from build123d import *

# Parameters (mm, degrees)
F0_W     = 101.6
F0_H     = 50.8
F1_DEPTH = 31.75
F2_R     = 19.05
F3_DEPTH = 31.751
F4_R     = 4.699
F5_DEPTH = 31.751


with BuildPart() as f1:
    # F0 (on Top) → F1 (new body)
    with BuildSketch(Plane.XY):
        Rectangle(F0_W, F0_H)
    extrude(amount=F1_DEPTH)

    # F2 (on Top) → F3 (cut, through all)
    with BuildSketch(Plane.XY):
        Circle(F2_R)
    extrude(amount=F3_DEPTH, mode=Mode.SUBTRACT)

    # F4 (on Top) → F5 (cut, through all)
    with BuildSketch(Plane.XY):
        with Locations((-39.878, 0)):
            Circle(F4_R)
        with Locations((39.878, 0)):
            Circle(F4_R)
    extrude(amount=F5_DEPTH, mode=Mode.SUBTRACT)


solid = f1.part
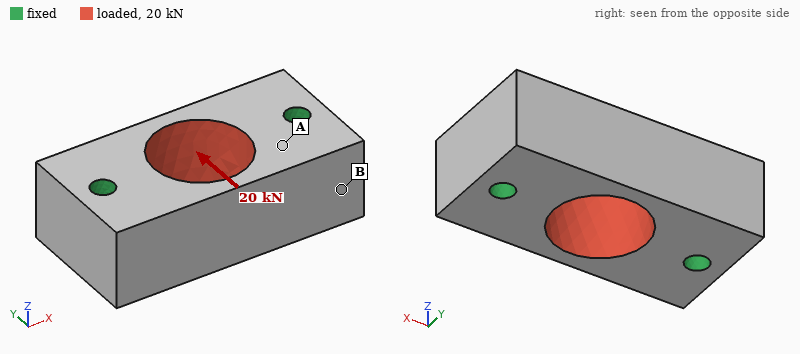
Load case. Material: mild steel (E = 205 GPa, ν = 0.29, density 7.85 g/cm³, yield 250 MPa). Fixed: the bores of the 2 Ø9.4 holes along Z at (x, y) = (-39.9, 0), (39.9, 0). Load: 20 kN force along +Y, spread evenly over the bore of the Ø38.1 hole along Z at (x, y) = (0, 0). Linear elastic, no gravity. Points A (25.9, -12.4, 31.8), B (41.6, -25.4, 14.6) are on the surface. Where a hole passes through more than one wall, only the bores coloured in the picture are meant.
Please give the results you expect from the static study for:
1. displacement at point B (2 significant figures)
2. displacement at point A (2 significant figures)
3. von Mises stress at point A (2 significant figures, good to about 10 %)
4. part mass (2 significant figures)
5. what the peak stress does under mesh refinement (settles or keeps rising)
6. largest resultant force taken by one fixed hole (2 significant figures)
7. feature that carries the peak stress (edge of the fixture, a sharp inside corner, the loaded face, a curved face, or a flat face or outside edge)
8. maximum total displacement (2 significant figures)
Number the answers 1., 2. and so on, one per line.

1. 2.1 µm
2. 2.3 µm
3. 14 MPa
4. 970 g
5. keeps rising
6. 10 kN
7. edge of the fixture
8. 6.5 µm
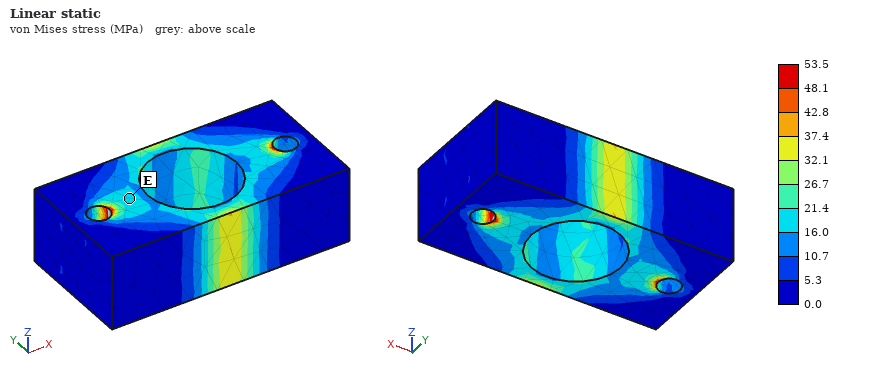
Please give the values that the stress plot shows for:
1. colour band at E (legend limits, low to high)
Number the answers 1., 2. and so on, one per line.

1. 16.0 to 21.4 MPa
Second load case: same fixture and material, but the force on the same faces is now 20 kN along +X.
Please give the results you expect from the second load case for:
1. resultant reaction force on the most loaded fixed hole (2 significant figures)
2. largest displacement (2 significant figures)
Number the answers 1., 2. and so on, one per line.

1. 10 kN
2. 2.3 µm
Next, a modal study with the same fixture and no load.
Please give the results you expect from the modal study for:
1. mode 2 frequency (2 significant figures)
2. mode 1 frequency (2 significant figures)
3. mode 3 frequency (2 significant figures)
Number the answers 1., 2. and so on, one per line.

1. 15 kHz
2. 13 kHz
3. 15 kHz
